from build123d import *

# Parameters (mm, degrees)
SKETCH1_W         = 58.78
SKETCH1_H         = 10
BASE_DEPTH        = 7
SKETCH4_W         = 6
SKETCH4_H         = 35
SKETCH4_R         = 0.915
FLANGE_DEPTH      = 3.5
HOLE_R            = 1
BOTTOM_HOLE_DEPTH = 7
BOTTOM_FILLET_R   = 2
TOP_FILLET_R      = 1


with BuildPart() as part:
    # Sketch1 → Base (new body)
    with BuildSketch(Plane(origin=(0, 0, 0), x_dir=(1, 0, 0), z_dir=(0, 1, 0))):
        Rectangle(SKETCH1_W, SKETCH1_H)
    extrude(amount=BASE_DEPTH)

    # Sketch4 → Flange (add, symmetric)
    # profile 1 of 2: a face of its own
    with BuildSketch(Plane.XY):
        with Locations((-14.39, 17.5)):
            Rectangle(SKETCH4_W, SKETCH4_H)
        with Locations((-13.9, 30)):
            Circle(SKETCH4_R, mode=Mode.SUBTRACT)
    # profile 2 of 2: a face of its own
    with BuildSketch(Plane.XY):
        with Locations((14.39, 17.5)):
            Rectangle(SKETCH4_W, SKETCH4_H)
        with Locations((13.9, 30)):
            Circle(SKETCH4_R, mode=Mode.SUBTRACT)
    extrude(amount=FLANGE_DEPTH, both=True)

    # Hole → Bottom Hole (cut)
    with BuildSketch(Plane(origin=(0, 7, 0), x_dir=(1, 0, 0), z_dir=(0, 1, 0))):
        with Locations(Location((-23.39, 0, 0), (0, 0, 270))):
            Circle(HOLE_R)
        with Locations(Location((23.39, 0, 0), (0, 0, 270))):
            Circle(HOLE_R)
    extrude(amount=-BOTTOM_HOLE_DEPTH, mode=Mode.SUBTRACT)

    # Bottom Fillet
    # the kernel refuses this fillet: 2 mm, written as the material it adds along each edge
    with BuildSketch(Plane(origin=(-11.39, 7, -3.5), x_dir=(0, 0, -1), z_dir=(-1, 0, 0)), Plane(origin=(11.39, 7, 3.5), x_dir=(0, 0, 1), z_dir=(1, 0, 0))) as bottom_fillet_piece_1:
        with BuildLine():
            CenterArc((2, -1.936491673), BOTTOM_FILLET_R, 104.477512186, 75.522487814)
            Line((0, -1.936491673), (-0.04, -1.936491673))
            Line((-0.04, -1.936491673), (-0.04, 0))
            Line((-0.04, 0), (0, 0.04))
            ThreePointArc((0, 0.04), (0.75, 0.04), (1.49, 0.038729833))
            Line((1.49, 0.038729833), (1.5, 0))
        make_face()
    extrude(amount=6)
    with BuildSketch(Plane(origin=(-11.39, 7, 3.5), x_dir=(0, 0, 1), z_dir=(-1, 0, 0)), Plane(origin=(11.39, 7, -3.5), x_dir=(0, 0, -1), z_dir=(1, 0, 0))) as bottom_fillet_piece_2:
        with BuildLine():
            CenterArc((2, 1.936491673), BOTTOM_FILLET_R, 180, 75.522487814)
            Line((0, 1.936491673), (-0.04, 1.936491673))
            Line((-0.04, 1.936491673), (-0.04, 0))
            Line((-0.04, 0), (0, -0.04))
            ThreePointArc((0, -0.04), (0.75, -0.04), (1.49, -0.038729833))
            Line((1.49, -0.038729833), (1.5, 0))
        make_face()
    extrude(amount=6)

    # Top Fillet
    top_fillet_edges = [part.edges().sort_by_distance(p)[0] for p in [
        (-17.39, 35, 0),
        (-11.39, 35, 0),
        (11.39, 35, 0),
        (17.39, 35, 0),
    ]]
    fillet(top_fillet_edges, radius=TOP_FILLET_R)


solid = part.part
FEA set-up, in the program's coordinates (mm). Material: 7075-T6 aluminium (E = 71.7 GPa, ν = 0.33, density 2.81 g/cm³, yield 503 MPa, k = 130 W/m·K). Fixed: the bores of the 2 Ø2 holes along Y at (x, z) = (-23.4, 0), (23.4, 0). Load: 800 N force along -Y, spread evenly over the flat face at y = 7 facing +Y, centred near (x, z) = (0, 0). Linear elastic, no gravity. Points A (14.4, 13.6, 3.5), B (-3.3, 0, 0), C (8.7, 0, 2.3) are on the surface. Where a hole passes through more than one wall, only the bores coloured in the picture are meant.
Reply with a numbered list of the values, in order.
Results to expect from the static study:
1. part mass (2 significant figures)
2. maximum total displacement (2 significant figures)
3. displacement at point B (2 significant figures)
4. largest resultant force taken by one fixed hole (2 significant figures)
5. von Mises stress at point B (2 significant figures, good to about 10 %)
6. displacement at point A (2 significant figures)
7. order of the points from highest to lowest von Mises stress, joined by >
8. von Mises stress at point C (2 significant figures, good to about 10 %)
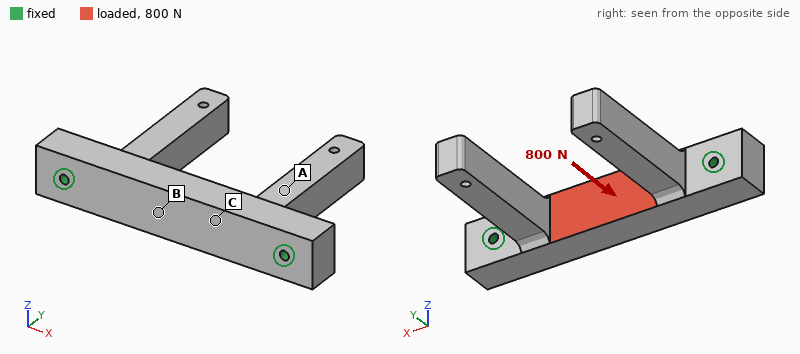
1. 18 g
2. 45 µm
3. 22 µm
4. 400 N
5. 33 MPa
6. 17 µm
7. B > C > A
8. 20 MPa
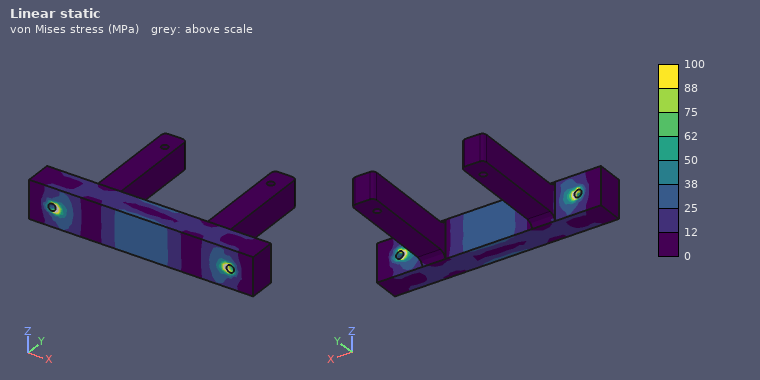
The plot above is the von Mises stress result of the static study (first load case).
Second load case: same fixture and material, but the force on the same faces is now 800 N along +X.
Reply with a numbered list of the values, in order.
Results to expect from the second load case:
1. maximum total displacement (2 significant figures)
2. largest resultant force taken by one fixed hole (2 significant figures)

1. 2.2 µm
2. 410 N
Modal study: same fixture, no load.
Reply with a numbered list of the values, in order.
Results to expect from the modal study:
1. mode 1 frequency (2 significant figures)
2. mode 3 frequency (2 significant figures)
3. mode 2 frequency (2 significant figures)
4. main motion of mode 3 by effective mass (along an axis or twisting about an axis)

1. 4700 Hz
2. 5400 Hz
3. 4700 Hz
4. along X
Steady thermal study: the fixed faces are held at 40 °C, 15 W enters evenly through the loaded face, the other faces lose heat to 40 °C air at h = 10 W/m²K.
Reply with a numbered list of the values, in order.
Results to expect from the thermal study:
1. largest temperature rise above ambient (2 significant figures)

1. 15 K
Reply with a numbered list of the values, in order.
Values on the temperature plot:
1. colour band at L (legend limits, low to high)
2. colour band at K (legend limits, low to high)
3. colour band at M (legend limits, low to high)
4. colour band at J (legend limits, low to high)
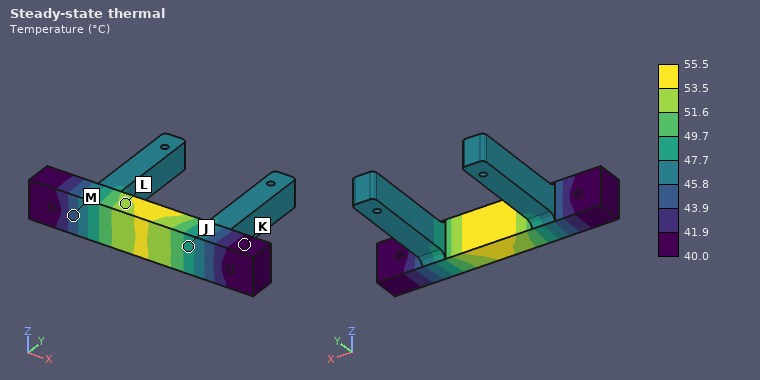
1. 51.6 to 53.5 °C
2. 40.0 to 41.9 °C
3. 43.9 to 45.8 °C
4. 47.7 to 49.7 °C
